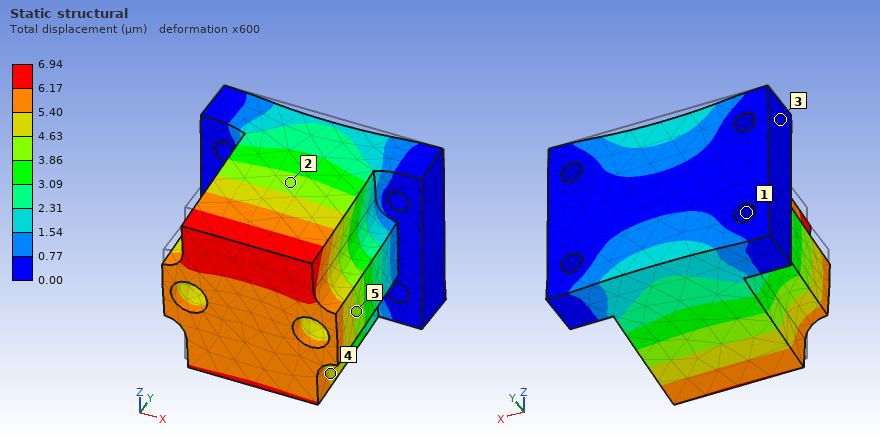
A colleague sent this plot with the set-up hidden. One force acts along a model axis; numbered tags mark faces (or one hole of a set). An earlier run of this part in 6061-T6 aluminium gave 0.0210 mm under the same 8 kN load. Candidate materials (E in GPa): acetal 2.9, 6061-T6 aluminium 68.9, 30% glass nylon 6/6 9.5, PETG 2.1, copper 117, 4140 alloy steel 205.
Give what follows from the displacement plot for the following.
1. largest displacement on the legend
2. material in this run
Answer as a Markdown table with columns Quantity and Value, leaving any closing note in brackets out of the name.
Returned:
| Quantity | Value |
|---|---|
| largest displacement on the legend | 6.94 µm |
| material in this run | 4140 alloy steel |
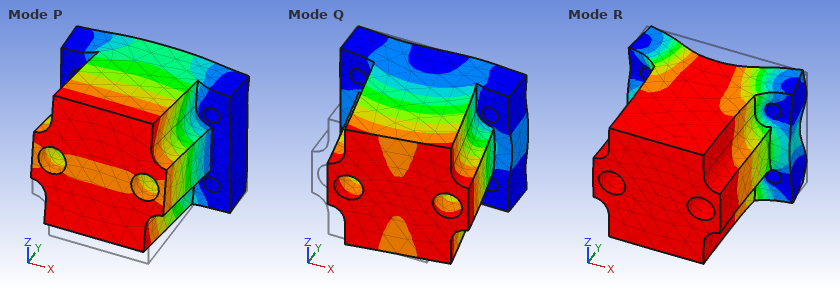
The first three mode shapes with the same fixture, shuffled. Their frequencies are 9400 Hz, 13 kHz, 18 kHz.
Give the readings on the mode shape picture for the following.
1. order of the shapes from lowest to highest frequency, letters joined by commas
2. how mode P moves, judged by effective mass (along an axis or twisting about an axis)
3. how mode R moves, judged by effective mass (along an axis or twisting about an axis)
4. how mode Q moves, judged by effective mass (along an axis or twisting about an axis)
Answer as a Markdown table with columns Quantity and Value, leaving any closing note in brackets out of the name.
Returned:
| Quantity | Value |
|---|---|
| order of the shapes from lowest to highest frequency, letters joined by commas | P, Q, R |
| how mode P moves, judged by effective mass | along Z |
| how mode R moves, judged by effective mass | along Y |
| how mode Q moves, judged by effective mass | along X |
